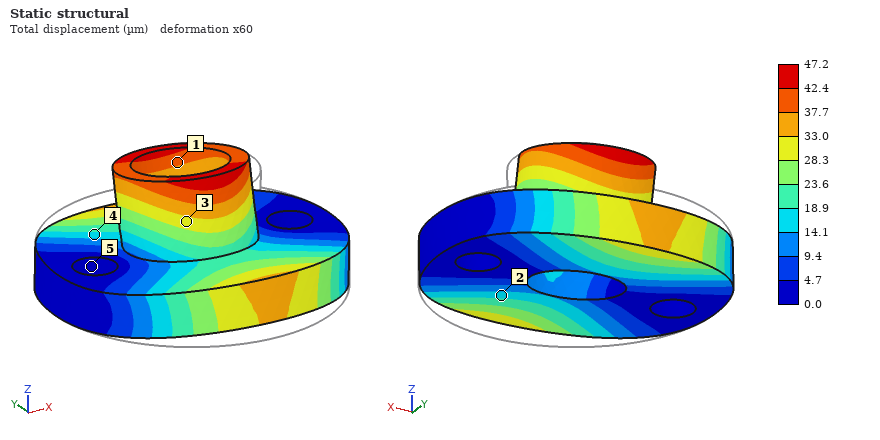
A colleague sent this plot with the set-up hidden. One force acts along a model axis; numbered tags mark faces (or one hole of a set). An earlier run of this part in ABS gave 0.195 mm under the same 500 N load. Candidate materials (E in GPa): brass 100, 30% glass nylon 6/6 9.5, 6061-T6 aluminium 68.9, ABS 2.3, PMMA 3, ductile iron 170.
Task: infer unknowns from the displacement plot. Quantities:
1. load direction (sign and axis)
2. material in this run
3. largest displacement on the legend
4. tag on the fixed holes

+Y
30% glass nylon 6/6
47.2 µm
5
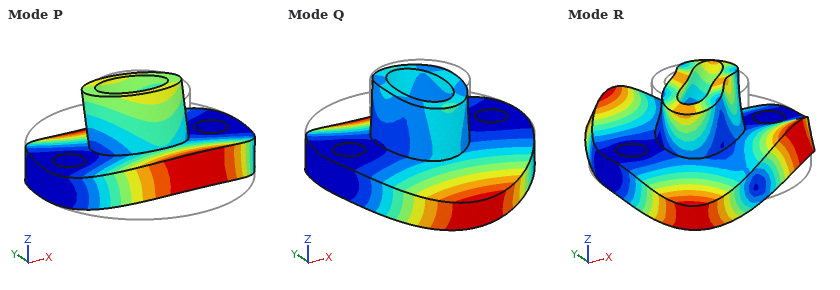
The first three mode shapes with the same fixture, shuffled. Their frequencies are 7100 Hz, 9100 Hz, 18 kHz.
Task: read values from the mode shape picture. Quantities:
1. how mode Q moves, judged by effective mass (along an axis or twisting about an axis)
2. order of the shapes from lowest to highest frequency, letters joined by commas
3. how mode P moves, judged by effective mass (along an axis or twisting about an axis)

along Z
P, Q, R
twisting about X
